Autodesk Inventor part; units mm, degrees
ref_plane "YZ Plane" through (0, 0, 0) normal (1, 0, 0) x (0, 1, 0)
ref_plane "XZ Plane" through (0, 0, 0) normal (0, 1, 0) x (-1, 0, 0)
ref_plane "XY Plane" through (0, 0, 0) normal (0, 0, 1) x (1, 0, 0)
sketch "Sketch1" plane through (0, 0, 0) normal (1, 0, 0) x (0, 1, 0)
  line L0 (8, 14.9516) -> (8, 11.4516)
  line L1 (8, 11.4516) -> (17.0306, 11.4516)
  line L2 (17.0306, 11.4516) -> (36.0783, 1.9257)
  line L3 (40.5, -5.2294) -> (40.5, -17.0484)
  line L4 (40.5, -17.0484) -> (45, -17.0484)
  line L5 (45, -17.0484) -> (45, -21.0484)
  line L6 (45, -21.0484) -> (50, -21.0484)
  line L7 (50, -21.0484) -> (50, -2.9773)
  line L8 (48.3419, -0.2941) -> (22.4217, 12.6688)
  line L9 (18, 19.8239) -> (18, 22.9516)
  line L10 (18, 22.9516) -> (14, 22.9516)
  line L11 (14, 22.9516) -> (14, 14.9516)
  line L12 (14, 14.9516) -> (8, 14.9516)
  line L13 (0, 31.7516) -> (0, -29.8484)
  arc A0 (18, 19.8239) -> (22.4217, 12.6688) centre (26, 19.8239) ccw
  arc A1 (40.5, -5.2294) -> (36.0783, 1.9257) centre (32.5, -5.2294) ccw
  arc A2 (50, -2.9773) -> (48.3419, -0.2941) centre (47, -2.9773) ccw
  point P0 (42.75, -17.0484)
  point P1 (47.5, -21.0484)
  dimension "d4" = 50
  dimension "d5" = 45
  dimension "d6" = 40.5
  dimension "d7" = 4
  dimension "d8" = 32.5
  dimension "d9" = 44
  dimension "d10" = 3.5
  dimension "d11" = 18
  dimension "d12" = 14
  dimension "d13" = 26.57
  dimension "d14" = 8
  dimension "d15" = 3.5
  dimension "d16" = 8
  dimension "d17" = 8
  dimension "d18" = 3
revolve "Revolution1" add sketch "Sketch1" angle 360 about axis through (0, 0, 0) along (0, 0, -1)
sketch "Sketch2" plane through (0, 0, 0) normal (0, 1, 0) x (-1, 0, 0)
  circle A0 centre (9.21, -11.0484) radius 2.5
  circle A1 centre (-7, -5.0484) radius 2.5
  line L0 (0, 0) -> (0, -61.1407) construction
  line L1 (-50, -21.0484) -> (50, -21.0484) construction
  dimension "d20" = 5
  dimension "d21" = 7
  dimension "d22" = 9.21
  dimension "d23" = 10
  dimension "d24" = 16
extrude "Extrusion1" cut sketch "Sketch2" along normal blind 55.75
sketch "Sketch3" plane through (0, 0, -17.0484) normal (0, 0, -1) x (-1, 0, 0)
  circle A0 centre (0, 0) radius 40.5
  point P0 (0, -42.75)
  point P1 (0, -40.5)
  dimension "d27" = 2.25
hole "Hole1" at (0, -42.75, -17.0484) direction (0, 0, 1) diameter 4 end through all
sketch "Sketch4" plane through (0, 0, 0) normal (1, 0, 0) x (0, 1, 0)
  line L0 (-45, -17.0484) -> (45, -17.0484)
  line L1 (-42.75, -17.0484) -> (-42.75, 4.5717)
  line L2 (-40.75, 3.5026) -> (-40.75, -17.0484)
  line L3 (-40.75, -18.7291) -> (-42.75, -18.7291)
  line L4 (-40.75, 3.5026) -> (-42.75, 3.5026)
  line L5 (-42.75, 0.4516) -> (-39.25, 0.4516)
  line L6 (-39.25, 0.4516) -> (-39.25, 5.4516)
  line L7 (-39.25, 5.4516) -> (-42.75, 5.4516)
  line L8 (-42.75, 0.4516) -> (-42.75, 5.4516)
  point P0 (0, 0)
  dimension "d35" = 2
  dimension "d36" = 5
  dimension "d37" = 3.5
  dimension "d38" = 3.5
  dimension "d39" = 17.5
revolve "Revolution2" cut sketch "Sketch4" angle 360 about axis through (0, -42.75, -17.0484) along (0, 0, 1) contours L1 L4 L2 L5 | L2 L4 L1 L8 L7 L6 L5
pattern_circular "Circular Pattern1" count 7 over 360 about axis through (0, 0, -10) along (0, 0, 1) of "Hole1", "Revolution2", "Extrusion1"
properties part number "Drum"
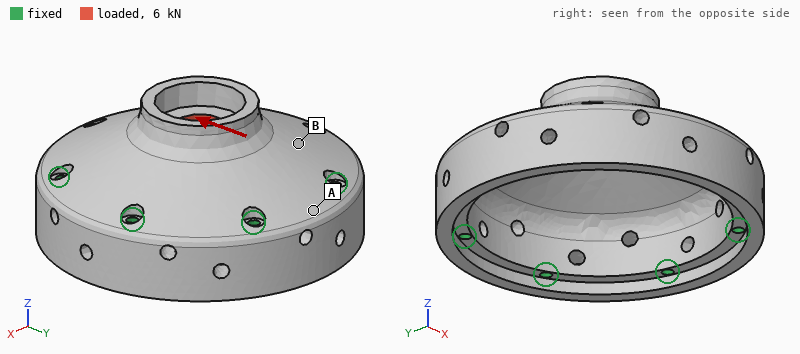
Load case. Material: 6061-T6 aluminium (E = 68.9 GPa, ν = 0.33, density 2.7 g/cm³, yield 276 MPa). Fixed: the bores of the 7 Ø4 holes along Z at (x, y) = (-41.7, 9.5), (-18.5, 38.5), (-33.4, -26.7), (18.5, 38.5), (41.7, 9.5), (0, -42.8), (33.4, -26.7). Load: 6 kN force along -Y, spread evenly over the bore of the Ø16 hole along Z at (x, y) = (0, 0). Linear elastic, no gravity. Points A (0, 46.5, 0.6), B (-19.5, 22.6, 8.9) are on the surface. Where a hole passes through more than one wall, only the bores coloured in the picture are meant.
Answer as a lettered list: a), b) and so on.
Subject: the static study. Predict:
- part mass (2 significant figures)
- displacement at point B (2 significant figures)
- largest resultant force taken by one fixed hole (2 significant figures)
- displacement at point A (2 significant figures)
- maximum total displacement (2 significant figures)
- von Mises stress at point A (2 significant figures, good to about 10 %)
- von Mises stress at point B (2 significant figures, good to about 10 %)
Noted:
a) 200 g
b) 10 µm
c) 1.1 kN
d) 4.0 µm
e) 21 µm
f) 6.8 MPa
g) 16 MPa
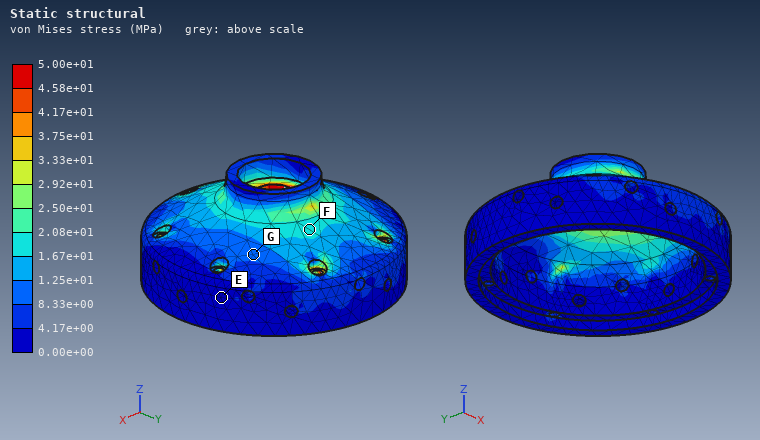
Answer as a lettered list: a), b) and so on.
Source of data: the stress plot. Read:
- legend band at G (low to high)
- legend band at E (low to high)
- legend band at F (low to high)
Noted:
a) 8.33e+00 to 1.25e+01 MPa
b) 0.00e+00 to 4.17e+00 MPa
c) 1.67e+01 to 2.08e+01 MPa
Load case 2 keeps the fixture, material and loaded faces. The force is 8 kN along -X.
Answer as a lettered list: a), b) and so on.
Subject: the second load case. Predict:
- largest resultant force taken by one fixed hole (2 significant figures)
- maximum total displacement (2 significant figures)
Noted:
a) 1.4 kN
b) 28 µm
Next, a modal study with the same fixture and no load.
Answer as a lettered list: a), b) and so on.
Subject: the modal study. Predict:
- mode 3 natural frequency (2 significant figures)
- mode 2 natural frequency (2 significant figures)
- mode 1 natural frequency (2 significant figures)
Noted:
a) 14 kHz
b) 14 kHz
c) 14 kHz
